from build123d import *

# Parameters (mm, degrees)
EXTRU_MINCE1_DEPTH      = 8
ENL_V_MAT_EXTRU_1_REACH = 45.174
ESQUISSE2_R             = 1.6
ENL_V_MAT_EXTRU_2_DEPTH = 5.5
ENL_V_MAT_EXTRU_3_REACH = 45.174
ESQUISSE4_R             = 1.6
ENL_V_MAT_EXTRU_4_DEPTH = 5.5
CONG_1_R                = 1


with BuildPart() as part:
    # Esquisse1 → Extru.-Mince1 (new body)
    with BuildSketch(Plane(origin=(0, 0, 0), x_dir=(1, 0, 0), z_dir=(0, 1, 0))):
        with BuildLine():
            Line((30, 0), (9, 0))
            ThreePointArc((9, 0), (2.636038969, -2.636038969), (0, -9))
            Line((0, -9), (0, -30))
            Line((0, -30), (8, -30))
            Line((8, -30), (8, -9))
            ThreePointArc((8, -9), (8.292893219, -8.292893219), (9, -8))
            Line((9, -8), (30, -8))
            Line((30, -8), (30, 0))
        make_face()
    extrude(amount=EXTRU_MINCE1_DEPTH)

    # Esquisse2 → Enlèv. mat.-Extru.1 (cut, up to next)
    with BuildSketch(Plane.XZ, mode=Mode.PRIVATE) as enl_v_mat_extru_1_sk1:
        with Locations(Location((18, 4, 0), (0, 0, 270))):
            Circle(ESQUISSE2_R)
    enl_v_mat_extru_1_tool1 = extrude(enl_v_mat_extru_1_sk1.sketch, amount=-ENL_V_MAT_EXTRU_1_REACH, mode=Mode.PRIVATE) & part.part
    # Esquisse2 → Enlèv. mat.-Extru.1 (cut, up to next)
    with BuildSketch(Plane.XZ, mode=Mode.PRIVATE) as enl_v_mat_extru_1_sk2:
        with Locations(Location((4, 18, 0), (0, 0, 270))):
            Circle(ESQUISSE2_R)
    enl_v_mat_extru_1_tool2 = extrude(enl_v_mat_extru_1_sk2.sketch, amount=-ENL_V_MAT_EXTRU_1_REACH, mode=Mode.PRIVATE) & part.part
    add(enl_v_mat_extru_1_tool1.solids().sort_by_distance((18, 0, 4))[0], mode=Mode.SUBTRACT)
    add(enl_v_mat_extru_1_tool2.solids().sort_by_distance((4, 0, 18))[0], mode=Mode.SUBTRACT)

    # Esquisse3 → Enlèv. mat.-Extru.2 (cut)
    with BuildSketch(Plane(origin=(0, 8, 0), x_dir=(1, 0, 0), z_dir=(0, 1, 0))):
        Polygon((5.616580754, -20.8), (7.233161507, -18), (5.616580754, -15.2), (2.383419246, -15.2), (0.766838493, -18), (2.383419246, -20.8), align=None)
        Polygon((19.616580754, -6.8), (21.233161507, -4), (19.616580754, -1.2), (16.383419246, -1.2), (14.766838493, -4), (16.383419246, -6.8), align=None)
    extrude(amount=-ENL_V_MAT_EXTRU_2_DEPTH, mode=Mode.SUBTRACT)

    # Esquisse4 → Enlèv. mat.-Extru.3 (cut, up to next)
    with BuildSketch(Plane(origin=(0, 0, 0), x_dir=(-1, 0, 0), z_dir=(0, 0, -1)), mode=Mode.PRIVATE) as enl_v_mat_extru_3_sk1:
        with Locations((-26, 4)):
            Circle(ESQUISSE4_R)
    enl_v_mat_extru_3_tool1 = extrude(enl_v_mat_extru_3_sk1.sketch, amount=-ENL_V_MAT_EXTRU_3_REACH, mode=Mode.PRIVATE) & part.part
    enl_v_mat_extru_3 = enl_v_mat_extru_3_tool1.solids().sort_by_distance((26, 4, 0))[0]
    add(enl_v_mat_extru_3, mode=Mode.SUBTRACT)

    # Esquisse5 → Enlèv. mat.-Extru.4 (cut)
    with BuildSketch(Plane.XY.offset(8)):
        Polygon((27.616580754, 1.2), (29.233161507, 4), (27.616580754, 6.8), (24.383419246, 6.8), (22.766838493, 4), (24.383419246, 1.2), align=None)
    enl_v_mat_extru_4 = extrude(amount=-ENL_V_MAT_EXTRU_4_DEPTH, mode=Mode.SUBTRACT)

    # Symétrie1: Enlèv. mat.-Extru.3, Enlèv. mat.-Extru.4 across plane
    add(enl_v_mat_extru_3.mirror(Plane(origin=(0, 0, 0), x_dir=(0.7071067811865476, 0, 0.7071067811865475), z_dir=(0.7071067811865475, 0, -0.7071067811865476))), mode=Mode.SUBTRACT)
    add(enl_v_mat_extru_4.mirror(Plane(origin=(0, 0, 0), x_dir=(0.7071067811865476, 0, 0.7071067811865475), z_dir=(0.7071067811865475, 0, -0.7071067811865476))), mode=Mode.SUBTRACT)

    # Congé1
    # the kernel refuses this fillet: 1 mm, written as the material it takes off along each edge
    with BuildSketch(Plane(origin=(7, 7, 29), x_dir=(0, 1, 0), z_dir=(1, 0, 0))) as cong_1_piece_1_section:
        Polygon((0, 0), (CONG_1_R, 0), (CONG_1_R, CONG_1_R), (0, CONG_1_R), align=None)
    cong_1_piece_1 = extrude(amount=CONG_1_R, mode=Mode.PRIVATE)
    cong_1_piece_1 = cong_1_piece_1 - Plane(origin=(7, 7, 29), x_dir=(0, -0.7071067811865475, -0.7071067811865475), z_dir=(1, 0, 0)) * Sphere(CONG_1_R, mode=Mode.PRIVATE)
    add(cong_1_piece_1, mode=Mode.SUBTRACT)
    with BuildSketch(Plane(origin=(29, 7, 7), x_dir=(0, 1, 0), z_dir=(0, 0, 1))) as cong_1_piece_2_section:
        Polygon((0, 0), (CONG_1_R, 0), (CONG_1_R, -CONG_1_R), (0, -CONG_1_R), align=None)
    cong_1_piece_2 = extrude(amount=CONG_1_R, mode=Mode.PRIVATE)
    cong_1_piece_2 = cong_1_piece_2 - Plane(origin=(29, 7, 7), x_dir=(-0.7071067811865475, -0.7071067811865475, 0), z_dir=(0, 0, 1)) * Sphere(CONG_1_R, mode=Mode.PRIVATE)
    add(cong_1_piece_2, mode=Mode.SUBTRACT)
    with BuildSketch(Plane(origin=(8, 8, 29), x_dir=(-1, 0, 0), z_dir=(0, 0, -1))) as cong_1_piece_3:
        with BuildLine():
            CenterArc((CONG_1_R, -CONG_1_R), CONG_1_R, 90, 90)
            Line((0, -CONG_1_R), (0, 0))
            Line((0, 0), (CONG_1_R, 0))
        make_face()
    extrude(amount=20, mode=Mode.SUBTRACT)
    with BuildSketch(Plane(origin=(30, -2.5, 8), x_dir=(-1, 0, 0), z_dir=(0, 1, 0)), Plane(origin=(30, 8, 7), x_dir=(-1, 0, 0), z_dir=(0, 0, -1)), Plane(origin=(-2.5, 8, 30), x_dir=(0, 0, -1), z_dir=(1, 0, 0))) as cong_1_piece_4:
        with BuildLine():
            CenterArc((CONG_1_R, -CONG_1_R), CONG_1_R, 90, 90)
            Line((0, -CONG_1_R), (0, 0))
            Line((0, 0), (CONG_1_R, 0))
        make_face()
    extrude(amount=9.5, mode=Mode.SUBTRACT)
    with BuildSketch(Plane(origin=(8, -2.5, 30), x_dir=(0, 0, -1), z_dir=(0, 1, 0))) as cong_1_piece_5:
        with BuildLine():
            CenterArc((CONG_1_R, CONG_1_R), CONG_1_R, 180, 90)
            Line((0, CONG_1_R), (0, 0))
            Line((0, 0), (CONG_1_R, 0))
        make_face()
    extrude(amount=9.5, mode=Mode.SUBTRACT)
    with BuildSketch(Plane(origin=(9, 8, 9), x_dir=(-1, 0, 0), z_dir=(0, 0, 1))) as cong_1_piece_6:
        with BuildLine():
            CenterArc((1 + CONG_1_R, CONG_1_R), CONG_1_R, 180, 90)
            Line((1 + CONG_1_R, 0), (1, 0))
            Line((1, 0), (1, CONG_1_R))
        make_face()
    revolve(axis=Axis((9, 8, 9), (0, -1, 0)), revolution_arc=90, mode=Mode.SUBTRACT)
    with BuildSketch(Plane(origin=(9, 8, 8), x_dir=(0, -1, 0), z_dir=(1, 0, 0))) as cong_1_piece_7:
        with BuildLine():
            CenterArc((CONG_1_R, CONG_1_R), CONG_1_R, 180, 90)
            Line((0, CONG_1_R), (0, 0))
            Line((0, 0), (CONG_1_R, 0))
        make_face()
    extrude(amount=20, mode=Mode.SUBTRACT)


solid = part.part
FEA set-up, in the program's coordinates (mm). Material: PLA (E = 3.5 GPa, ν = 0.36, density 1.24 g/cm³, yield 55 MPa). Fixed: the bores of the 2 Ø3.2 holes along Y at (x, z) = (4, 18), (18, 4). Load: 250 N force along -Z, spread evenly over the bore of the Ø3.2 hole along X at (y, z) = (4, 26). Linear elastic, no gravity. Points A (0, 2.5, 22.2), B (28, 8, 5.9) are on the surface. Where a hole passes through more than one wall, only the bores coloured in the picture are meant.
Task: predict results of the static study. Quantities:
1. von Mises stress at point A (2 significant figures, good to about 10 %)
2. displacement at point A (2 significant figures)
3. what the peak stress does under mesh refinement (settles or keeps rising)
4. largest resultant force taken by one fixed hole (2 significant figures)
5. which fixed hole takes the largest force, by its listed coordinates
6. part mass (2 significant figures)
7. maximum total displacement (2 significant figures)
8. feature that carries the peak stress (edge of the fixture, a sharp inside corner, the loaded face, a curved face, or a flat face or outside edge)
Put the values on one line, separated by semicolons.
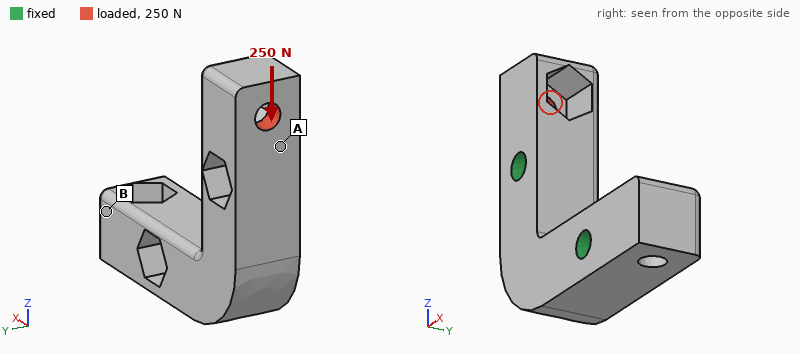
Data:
16 MPa; 0.049 mm; keeps rising; 240 N; (4, 18); 3.1 g; 0.15 mm; edge of the fixture
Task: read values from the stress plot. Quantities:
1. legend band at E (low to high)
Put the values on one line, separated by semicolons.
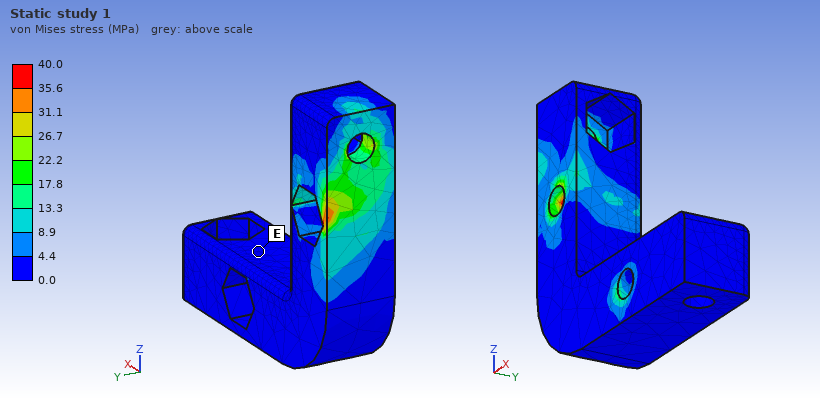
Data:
0.0 to 4.4 MPa
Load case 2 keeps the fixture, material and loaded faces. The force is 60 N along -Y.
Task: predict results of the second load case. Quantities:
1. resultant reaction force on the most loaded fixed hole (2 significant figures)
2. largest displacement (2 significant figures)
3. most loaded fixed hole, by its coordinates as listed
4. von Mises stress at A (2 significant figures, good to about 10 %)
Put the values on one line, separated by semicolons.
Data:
73 N; 0.10 mm; (4, 18); 5.7 MPa
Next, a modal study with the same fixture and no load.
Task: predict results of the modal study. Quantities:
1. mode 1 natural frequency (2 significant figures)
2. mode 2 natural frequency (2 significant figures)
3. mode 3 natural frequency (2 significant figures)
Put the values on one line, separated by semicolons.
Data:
4400 Hz; 7100 Hz; 7700 Hz
